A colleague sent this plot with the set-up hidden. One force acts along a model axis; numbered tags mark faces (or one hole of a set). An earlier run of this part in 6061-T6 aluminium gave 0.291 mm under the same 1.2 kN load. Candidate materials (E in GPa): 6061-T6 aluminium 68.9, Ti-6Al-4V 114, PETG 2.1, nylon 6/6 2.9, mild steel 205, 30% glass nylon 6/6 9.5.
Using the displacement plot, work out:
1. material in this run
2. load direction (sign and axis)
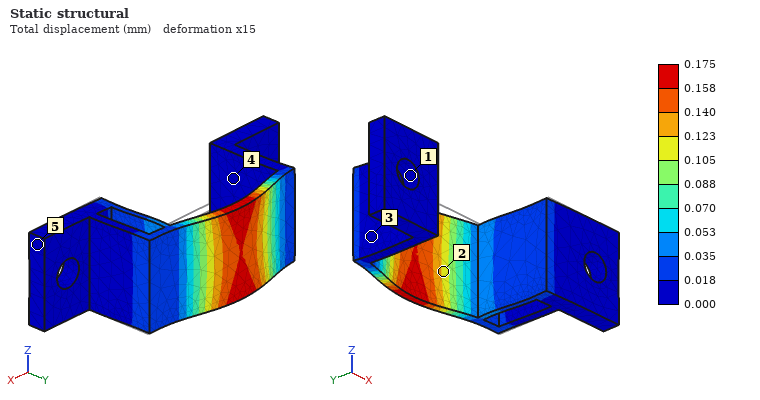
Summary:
Ti-6Al-4V
+Y
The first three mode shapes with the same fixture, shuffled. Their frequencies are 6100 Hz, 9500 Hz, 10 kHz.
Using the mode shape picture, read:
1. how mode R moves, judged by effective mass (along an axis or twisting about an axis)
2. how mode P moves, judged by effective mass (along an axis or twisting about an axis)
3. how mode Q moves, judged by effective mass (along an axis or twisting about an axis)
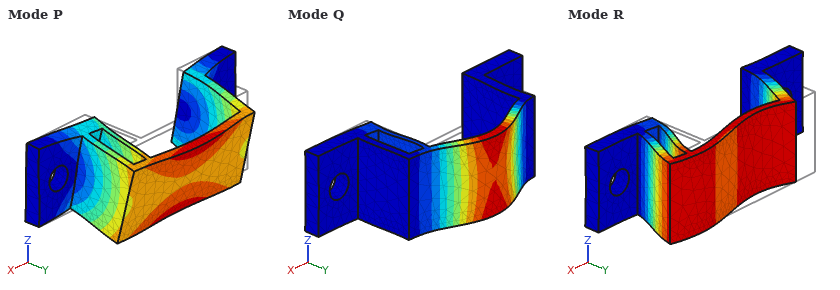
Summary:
along X
along Z
along Y
